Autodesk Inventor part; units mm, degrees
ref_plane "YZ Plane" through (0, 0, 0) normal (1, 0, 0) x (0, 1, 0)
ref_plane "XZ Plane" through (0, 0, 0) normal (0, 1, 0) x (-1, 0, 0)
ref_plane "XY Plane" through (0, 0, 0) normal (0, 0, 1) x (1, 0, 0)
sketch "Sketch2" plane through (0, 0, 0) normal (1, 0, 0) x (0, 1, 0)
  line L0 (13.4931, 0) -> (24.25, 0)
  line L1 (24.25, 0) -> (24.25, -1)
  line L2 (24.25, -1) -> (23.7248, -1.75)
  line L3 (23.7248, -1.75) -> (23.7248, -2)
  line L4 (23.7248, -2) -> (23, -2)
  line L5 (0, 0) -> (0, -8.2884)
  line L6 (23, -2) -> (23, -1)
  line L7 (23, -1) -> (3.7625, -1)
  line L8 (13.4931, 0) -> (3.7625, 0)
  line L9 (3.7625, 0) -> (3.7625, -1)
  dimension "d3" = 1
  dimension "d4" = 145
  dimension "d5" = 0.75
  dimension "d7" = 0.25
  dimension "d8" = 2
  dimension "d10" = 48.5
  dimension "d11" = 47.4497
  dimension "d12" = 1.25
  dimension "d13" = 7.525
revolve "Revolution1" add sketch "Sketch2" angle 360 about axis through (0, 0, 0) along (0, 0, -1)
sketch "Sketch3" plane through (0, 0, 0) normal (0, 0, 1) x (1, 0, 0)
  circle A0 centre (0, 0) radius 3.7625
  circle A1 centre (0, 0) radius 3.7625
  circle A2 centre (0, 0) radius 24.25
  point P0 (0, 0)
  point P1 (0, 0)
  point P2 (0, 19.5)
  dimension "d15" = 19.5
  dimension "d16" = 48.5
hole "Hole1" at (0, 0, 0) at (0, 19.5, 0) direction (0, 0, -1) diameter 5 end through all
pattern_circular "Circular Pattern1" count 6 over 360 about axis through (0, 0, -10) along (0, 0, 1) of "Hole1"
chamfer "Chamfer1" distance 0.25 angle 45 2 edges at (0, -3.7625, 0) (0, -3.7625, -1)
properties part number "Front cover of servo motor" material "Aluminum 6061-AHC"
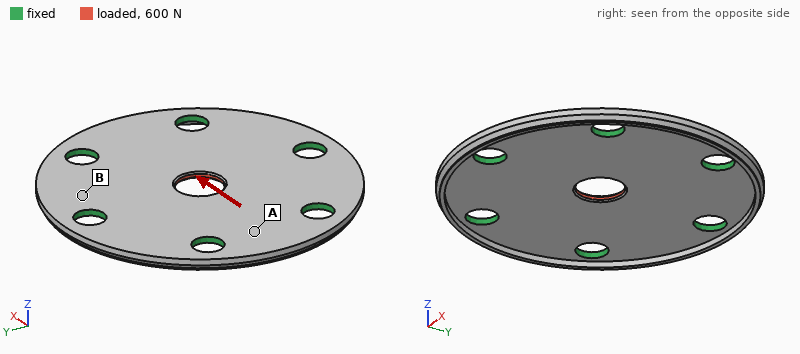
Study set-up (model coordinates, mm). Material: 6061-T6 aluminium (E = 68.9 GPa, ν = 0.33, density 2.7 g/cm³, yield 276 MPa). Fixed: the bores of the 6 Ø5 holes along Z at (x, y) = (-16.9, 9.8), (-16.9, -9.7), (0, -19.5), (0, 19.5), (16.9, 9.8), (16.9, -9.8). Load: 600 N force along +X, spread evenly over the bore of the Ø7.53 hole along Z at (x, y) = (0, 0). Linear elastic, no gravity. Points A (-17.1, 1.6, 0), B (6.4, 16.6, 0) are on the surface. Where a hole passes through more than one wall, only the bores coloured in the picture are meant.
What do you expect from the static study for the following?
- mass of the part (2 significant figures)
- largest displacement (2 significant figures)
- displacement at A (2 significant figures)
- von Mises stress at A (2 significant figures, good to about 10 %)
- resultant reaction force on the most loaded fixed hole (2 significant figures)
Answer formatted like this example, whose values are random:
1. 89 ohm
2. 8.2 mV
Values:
1. 4.9 g
2. 4.1 µm
3. 1.2 µm
4. 5.0 MPa
5. 140 N
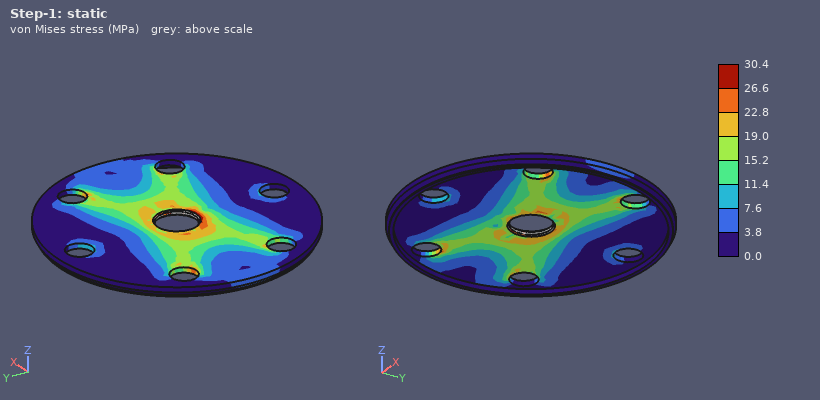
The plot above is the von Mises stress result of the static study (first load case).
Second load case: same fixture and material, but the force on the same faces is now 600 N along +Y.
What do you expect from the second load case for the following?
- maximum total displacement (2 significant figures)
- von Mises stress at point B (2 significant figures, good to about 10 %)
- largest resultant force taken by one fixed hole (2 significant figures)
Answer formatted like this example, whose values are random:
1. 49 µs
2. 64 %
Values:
1. 4.1 µm
2. 5.1 MPa
3. 160 N
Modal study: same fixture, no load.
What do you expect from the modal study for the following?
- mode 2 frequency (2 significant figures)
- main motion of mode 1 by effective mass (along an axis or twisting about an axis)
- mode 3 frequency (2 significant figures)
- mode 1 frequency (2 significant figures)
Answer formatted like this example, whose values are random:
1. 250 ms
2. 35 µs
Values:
1. 14 kHz
2. along Z
3. 14 kHz
4. 7400 Hz
